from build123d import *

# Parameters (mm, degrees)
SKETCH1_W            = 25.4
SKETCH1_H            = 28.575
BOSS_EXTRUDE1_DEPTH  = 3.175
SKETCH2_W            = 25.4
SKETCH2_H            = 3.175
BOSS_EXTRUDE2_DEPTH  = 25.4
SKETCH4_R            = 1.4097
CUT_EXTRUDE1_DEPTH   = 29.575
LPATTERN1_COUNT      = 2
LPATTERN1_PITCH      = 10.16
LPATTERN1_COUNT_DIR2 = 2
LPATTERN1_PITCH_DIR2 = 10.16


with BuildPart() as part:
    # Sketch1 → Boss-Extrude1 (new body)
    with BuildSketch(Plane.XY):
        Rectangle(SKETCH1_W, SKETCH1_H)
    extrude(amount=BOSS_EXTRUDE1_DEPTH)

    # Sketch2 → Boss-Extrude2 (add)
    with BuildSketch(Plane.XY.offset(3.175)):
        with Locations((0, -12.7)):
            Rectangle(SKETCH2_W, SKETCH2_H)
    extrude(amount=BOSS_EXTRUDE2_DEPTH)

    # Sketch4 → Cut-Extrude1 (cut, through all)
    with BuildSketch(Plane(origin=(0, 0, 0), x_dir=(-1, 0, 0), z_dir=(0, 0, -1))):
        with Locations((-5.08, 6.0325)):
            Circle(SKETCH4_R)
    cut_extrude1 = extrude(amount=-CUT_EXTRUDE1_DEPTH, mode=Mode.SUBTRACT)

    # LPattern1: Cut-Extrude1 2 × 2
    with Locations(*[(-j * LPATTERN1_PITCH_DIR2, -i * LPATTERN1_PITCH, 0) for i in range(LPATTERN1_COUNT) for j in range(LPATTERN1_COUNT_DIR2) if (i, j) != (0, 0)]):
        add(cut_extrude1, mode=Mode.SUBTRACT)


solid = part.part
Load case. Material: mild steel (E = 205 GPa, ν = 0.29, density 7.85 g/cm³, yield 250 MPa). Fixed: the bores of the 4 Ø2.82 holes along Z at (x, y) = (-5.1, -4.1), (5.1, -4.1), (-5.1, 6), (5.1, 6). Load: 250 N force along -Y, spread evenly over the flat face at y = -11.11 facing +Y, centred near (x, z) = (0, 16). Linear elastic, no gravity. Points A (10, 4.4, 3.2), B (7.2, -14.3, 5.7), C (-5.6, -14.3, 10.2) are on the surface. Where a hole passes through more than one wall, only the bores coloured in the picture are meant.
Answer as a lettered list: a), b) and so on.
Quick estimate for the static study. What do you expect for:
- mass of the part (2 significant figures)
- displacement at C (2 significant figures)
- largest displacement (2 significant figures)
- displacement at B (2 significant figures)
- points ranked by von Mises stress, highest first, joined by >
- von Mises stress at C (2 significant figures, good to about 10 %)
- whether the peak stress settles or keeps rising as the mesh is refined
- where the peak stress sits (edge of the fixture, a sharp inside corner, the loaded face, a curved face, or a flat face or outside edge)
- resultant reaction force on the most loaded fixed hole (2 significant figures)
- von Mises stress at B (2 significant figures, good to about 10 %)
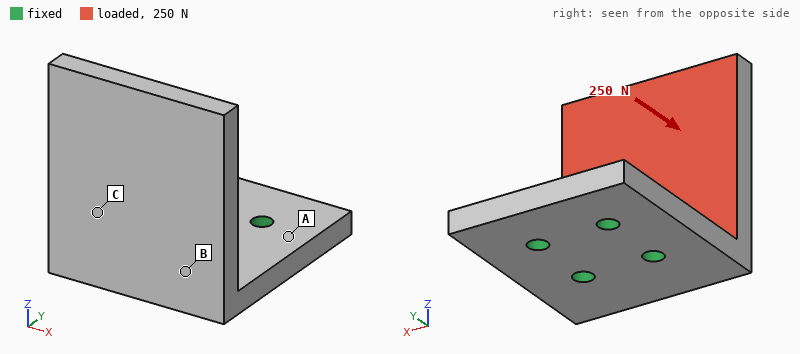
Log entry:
a) 34 g
b) 27 µm
c) 96 µm
d) 17 µm
e) B > C > A
f) 36 MPa
g) keeps rising
h) edge of the fixture
i) 120 N
j) 56 MPa
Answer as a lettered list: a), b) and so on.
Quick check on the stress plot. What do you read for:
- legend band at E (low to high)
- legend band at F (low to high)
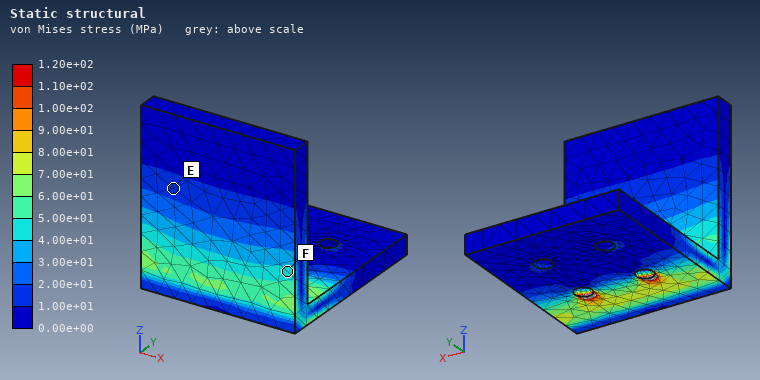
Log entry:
a) 1.00e+01 to 2.00e+01 MPa
b) 4.00e+01 to 5.00e+01 MPa
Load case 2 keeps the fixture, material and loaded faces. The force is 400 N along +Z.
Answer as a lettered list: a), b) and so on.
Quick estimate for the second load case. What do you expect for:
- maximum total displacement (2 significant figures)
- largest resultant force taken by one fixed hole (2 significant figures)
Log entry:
a) 9.5 µm
b) 230 N
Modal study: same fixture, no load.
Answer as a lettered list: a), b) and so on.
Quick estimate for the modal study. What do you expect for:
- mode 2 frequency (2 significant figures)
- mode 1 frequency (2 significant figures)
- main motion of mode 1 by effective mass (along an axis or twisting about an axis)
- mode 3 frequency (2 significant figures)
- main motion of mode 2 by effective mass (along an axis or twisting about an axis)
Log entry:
a) 5200 Hz
b) 2500 Hz
c) along Y
d) 8600 Hz
e) along X
